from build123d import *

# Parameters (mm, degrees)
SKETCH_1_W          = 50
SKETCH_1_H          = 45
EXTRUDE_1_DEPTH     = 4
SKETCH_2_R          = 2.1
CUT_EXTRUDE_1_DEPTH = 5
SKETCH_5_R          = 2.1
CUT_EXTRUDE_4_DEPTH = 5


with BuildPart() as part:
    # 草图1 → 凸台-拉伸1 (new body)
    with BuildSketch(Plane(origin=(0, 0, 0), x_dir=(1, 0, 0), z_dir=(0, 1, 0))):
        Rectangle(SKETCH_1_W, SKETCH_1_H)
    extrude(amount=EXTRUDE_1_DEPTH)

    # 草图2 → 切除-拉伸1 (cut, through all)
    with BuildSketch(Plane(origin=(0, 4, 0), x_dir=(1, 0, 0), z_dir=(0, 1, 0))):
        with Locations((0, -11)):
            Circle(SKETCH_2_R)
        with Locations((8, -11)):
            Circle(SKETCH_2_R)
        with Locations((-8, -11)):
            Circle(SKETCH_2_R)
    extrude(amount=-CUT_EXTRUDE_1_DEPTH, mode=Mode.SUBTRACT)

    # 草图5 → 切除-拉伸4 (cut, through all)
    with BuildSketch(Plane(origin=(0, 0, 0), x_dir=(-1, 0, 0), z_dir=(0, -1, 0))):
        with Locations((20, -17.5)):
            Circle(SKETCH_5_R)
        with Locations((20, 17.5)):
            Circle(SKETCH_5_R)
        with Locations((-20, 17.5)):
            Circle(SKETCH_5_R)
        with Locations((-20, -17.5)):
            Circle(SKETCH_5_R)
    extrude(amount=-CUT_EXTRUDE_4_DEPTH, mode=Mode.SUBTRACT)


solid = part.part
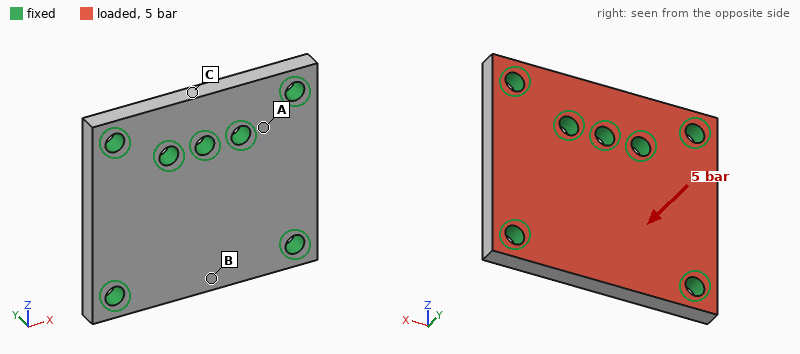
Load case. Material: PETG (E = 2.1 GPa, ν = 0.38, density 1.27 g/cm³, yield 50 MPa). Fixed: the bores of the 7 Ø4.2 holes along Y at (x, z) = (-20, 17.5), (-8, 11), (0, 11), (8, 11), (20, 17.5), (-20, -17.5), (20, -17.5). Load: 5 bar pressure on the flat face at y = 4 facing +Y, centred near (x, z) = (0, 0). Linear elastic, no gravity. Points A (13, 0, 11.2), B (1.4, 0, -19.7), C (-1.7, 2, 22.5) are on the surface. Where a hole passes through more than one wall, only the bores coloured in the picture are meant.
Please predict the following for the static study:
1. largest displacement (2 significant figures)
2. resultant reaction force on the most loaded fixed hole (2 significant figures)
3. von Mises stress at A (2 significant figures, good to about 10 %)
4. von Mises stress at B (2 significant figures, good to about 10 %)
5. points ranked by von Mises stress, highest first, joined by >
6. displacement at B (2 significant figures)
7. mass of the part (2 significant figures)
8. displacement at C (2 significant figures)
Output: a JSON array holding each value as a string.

["0.29 mm", "220 N", "6.1 MPa", "11 MPa", "B > A > C", "0.27 mm", "11 g", "0.045 mm"]
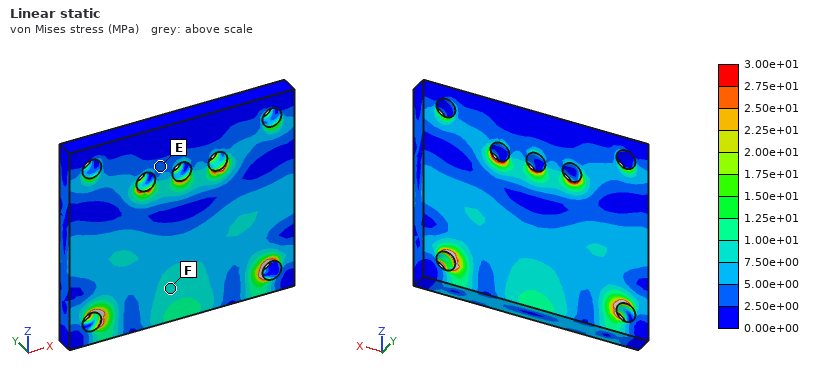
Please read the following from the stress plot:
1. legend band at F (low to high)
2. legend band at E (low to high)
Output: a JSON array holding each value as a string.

["7.50e+00 to 1.00e+01 MPa", "2.50e+00 to 5.00e+00 MPa"]
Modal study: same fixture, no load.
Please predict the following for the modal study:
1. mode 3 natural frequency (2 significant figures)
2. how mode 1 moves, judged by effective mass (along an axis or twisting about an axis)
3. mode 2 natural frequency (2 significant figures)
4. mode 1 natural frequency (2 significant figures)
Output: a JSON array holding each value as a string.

["5300 Hz", "along Y", "5200 Hz", "3600 Hz"]
